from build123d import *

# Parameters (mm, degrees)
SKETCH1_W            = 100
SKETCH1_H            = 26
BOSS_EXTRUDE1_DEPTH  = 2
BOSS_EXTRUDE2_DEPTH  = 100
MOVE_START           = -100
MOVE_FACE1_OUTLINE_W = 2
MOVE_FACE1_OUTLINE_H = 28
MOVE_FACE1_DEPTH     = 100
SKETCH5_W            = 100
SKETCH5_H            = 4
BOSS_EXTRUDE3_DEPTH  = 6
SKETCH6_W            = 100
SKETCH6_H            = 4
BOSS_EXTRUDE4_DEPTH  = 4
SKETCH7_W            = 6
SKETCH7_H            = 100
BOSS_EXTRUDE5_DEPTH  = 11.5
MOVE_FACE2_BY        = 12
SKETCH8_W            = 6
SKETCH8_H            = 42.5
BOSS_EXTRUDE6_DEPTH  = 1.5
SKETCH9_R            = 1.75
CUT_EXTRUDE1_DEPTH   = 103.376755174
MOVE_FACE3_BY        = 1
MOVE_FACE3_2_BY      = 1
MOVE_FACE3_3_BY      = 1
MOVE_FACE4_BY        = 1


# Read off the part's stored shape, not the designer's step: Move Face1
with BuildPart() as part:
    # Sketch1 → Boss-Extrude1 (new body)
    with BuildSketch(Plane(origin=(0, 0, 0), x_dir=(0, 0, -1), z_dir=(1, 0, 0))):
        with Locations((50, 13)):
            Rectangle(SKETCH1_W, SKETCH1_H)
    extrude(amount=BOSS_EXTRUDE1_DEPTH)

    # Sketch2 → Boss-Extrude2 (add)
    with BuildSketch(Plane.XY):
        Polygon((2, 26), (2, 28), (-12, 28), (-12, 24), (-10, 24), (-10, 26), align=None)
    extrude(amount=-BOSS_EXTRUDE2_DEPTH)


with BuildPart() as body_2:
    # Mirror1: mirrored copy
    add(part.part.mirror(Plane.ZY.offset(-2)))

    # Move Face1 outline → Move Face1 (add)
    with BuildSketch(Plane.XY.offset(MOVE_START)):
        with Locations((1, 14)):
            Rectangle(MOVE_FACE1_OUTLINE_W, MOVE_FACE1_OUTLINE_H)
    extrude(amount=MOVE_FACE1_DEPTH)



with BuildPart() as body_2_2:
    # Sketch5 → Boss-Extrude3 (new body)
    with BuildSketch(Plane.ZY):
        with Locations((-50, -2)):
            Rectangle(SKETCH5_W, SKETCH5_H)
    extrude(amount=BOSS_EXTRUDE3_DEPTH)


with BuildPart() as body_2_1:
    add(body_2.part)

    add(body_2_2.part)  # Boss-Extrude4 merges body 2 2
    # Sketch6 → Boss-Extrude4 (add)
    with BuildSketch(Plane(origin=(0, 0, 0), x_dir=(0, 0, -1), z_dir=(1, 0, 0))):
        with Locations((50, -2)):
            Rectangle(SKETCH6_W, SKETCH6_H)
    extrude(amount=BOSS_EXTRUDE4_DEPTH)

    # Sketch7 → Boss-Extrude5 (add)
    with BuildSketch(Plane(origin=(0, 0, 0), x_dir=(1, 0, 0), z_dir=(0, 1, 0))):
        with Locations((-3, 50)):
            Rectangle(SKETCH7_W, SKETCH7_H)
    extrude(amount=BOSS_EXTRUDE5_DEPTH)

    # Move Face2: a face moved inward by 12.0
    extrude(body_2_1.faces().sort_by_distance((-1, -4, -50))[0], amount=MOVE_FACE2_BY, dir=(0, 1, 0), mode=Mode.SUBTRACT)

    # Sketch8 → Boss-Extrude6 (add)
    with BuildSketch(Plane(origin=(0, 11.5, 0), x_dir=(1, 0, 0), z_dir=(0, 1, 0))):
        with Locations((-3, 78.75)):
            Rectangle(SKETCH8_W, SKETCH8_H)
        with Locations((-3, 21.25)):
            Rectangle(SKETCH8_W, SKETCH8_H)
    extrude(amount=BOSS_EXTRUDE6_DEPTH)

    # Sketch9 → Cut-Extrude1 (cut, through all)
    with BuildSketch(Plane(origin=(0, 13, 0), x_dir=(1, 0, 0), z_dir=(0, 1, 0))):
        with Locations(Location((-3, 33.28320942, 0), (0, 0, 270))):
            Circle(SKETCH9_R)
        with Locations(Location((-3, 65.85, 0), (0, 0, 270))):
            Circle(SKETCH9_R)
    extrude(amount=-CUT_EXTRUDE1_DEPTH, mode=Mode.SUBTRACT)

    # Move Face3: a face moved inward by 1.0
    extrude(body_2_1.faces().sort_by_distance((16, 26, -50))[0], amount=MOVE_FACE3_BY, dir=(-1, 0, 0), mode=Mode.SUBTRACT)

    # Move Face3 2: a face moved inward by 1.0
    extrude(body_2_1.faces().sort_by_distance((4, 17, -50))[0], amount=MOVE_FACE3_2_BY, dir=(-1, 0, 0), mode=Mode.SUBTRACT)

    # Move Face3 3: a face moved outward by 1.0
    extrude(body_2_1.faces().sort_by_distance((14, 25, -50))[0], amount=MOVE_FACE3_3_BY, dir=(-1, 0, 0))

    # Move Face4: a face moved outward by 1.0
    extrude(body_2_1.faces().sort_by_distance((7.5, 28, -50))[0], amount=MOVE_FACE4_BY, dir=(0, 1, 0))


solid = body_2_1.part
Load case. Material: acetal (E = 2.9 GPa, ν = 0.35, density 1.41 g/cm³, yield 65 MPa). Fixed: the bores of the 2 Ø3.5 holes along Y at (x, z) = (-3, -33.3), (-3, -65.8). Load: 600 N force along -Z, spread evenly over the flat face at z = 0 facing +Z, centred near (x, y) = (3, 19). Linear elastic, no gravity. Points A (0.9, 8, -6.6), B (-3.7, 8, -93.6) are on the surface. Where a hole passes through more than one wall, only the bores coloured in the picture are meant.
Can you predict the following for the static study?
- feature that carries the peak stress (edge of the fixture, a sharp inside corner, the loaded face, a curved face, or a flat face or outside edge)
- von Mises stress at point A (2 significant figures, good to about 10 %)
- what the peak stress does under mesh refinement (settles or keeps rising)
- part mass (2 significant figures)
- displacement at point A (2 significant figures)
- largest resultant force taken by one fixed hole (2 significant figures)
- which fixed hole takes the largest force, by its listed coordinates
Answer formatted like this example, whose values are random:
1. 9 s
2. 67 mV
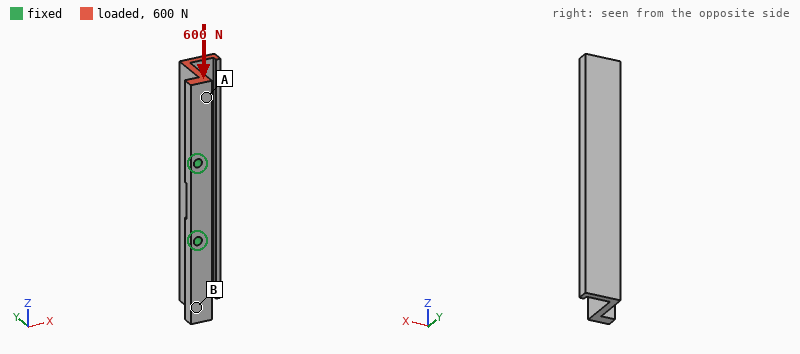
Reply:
1. edge of the fixture
2. 4.6 MPa
3. keeps rising
4. 18 g
5. 0.18 mm
6. 440 N
7. (-3, -33.3)
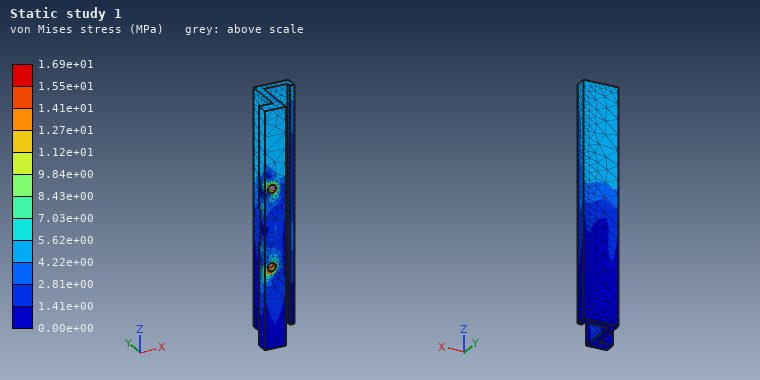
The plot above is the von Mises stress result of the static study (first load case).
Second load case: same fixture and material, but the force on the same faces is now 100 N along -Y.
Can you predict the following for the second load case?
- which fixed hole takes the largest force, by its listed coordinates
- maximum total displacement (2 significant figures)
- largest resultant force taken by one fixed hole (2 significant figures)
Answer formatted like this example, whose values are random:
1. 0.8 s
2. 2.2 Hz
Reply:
1. (-3, -33.3)
2. 0.91 mm
3. 200 N
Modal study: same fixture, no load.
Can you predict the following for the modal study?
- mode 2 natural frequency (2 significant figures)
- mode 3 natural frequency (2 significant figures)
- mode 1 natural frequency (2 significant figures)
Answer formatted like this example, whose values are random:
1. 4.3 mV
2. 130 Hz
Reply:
1. 730 Hz
2. 1500 Hz
3. 720 Hz
